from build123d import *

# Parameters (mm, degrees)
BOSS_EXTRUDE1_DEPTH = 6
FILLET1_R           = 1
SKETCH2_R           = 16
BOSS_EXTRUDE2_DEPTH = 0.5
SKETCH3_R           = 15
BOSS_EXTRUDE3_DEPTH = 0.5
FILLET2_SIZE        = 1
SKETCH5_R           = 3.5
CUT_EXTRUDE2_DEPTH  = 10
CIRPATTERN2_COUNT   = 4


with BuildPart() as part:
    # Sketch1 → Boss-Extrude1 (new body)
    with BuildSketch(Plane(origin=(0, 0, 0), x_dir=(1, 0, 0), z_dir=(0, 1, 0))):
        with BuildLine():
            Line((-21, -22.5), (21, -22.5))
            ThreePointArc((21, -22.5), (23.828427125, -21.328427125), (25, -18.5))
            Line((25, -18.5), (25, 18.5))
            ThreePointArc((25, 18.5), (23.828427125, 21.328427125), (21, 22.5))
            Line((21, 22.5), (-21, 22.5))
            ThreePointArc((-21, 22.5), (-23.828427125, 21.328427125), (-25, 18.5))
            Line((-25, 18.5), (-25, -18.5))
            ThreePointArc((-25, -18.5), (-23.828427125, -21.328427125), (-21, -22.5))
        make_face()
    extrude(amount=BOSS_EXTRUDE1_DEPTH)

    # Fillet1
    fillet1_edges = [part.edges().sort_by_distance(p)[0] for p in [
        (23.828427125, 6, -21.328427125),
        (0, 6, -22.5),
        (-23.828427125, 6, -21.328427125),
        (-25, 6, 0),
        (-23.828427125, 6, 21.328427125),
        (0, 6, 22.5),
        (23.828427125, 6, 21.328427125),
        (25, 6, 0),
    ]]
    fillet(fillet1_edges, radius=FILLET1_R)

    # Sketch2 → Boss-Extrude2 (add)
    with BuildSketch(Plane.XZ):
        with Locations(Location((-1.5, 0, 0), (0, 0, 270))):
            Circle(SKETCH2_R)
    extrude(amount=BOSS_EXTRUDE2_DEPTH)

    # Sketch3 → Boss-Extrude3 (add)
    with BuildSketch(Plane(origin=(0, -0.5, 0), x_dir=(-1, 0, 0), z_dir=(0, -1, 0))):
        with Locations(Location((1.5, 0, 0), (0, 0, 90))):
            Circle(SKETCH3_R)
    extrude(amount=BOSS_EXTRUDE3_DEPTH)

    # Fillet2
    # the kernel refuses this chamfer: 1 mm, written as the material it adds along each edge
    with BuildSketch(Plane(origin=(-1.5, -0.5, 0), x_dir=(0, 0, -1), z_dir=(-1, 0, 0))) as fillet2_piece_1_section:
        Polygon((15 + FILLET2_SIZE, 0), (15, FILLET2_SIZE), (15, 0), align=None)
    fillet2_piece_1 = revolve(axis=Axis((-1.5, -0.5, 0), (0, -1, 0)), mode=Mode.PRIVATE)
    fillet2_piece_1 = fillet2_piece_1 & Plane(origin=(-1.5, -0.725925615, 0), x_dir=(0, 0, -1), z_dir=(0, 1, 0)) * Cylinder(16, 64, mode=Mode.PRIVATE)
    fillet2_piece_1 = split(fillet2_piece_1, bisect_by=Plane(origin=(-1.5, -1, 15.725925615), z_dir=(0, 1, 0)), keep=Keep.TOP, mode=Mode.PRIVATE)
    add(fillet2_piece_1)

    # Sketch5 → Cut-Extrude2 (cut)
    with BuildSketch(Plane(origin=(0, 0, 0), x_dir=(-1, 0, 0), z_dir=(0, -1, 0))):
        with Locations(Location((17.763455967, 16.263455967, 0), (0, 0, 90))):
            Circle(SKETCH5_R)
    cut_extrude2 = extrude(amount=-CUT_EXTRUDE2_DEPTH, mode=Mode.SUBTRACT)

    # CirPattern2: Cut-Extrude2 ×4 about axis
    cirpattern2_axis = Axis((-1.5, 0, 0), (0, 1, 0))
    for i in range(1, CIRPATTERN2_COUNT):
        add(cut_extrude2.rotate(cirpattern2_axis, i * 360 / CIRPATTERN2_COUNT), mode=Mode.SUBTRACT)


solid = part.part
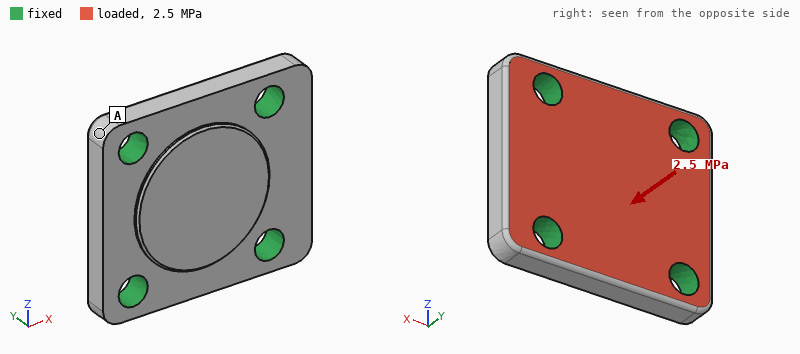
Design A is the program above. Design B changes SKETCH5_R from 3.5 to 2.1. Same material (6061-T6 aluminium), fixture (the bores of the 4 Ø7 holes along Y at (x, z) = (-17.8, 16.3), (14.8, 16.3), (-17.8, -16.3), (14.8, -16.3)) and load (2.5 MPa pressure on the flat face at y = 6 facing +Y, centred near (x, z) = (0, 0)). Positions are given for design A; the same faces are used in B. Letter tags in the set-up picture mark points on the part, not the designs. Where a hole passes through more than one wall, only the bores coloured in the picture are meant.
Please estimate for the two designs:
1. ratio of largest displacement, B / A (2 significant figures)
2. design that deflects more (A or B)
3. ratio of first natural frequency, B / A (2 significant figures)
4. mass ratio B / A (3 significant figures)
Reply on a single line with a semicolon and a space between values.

1.4; B; 0.83; 1.04
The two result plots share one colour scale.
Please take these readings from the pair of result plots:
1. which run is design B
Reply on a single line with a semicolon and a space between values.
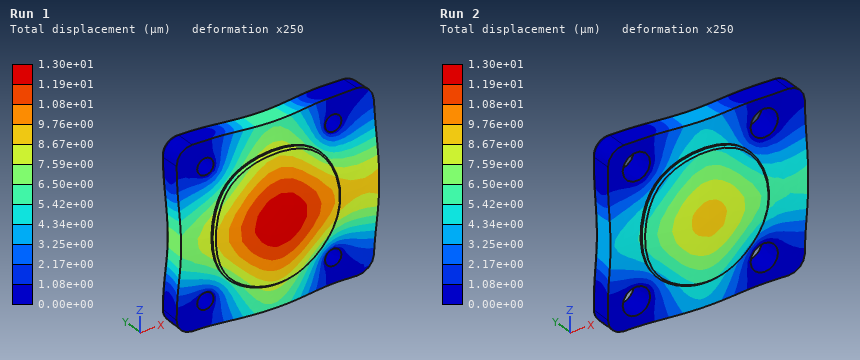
Run 1
